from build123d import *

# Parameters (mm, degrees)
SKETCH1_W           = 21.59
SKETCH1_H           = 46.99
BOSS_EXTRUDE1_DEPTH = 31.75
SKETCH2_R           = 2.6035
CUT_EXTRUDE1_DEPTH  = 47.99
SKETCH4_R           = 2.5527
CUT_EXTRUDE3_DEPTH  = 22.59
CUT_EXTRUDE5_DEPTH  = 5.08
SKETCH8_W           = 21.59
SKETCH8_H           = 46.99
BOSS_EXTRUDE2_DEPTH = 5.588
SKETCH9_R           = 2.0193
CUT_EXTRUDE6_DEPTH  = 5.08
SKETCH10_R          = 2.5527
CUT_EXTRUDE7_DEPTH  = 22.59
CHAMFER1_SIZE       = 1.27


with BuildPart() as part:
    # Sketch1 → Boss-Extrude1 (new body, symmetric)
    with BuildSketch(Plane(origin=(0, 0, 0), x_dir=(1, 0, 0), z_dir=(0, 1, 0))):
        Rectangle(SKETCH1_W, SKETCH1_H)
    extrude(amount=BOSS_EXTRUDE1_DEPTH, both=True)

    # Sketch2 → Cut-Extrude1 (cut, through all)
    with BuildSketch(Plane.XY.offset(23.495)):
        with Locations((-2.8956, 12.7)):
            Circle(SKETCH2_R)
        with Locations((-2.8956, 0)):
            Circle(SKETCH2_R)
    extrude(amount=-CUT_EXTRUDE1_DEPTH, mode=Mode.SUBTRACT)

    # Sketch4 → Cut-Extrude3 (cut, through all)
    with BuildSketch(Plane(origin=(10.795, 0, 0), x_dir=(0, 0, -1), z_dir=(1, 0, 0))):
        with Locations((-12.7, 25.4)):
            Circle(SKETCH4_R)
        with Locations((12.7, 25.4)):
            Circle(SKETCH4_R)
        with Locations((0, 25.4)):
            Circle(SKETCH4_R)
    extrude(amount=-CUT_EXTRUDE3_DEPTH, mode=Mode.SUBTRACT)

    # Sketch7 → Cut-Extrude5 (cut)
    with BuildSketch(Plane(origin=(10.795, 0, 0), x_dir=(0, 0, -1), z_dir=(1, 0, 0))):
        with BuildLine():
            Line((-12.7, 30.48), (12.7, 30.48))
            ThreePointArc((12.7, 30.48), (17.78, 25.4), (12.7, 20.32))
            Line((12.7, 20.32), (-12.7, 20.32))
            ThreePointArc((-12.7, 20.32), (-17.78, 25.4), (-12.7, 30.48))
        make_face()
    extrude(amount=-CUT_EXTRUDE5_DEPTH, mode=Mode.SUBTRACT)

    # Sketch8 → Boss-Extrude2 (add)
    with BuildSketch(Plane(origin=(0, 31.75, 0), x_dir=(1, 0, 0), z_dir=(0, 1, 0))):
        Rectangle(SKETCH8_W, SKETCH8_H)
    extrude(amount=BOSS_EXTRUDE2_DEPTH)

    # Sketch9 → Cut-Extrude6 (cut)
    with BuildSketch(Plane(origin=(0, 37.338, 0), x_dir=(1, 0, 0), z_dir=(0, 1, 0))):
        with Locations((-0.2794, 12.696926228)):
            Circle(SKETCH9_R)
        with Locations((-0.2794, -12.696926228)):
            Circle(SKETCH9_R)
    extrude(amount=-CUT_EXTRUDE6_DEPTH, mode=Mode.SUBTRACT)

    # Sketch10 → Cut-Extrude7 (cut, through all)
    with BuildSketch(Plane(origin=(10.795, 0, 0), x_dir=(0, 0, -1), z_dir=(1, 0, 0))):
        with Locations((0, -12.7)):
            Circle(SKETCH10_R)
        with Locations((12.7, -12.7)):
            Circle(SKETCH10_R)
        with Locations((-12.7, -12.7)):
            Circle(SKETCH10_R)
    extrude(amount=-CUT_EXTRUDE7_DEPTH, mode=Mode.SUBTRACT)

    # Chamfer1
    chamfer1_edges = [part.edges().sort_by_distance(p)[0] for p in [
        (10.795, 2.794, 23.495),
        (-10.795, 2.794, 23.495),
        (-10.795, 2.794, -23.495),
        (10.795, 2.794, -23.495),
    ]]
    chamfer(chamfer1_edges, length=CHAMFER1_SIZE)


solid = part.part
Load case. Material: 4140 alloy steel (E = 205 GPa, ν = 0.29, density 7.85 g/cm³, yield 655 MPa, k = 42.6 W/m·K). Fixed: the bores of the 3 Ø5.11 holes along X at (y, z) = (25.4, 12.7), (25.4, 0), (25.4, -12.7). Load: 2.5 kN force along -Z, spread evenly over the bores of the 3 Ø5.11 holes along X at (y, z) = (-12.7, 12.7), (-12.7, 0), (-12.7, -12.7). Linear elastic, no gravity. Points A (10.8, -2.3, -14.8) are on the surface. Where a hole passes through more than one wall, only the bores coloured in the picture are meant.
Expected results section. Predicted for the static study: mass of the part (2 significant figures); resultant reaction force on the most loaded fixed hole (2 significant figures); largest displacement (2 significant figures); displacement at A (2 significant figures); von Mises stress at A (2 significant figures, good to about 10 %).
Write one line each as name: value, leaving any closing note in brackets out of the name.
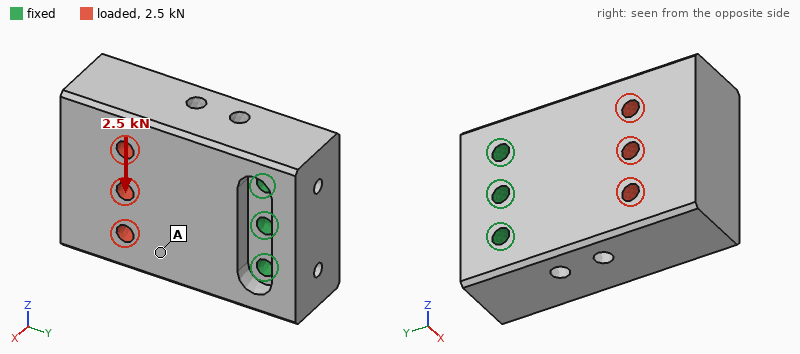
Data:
mass of the part: 500 g
resultant reaction force on the most loaded fixed hole: 3.3 kN
largest displacement: 6.0 µm
displacement at A: 2.8 µm
von Mises stress at A: 4.8 MPa
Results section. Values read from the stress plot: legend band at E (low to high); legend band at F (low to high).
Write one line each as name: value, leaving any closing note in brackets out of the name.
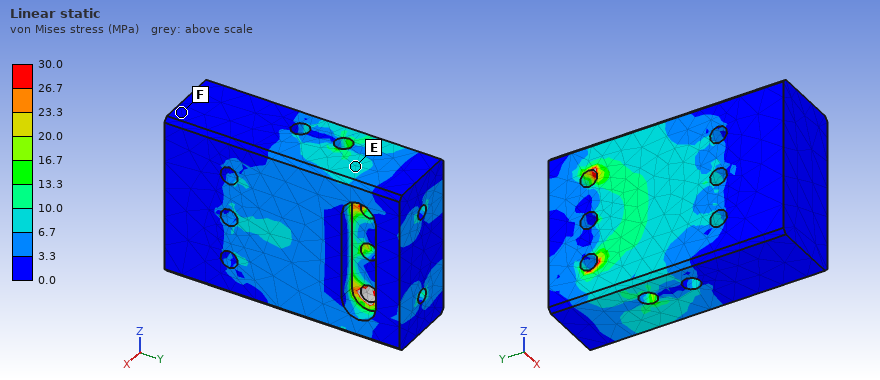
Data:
legend band at E: 6.7 to 10.0 MPa
legend band at F: 0.0 to 3.3 MPa
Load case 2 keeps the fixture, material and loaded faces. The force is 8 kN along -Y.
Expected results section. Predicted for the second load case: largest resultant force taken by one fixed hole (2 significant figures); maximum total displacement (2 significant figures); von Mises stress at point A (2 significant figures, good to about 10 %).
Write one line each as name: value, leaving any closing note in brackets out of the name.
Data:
largest resultant force taken by one fixed hole: 3.0 kN
maximum total displacement: 3.2 µm
von Mises stress at point A: 7.9 MPa
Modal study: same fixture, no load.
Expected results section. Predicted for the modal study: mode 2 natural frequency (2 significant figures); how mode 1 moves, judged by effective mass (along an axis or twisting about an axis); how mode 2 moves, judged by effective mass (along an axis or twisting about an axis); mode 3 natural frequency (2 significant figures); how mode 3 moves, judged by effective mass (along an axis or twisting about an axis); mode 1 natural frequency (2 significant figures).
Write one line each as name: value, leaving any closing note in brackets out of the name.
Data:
mode 2 natural frequency: 6800 Hz
how mode 1 moves, judged by effective mass: along X
how mode 2 moves, judged by effective mass: along Z
mode 3 natural frequency: 9500 Hz
how mode 3 moves, judged by effective mass: twisting about Y
mode 1 natural frequency: 4000 Hz
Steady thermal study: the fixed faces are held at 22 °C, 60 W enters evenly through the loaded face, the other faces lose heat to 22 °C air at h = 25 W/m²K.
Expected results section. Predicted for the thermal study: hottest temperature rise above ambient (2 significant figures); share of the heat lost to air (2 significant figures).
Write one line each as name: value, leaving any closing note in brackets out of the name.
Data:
hottest temperature rise above ambient: 59 K
share of the heat lost to air: 16 %
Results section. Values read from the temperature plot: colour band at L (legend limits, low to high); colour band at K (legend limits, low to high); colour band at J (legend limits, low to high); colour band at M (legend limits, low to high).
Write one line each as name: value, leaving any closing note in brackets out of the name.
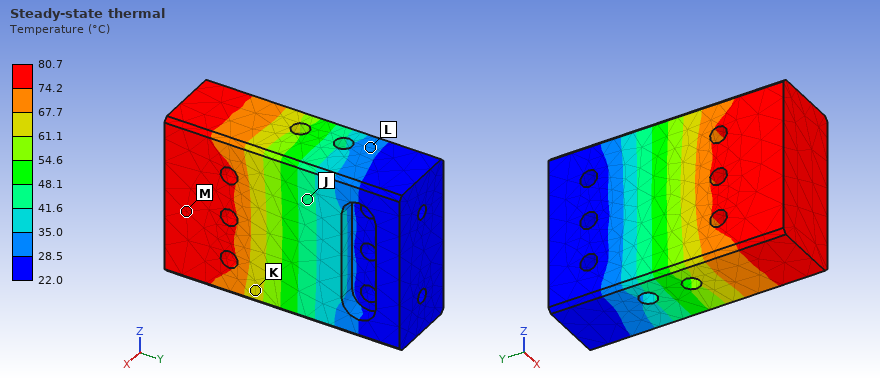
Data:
colour band at L: 28.5 to 35.0 °C
colour band at K: 61.1 to 67.7 °C
colour band at J: 41.6 to 48.1 °C
colour band at M: 74.2 to 80.7 °C
